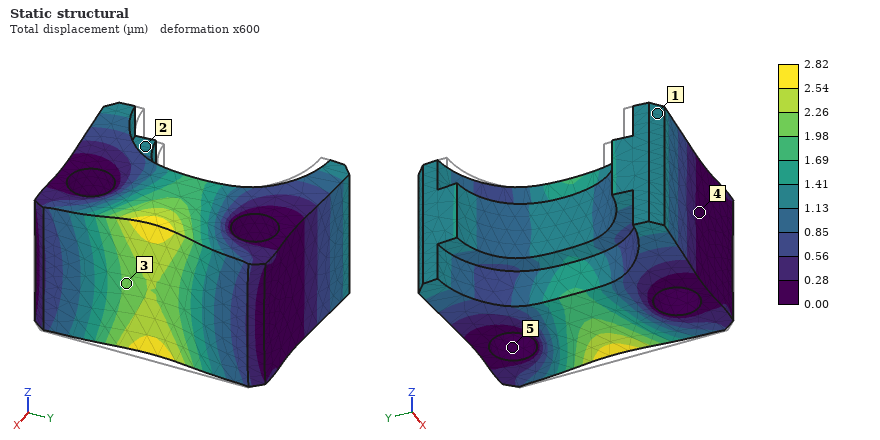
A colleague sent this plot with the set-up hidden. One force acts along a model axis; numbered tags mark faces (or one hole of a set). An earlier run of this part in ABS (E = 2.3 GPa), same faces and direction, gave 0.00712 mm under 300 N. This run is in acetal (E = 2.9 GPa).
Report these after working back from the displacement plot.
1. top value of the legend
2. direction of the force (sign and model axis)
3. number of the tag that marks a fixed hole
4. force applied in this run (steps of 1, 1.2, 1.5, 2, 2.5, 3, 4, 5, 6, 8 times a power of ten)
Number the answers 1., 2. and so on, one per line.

1. 2.82 µm
2. -X
3. 5
4. 150 N
